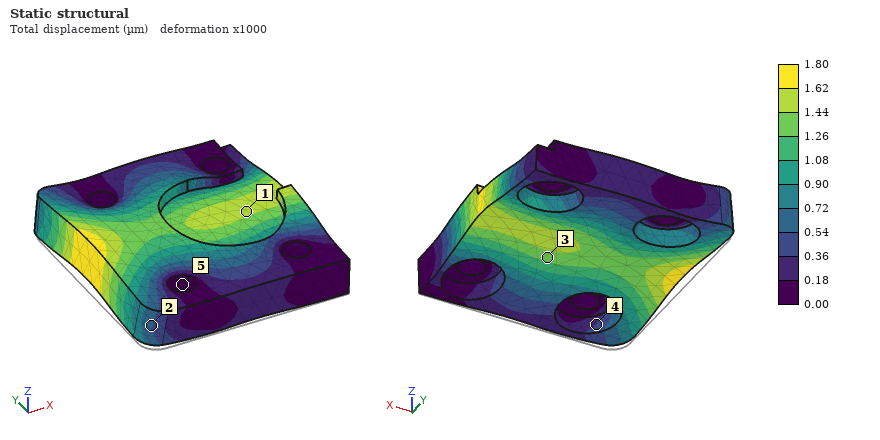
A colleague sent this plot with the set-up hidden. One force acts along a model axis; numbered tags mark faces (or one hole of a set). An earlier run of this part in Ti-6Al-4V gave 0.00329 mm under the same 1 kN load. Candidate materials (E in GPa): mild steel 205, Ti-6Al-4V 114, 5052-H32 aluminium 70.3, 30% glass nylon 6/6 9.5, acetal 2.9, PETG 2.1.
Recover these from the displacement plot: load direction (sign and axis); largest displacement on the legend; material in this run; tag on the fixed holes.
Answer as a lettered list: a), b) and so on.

a) +Z
b) 1.80 µm
c) mild steel
d) 5
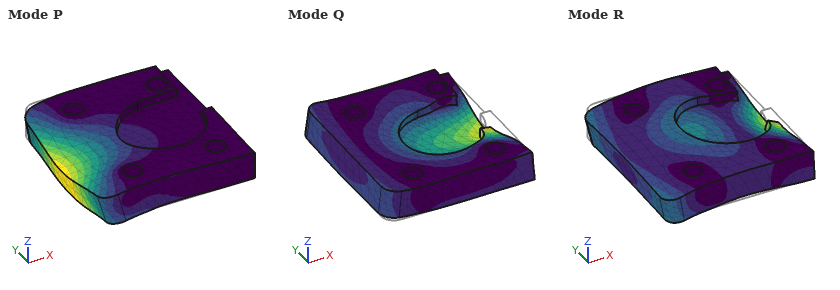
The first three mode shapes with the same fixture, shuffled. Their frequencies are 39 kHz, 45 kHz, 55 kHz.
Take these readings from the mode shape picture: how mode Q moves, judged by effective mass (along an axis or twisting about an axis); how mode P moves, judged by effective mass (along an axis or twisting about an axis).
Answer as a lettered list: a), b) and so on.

a) along Z
b) along Z
